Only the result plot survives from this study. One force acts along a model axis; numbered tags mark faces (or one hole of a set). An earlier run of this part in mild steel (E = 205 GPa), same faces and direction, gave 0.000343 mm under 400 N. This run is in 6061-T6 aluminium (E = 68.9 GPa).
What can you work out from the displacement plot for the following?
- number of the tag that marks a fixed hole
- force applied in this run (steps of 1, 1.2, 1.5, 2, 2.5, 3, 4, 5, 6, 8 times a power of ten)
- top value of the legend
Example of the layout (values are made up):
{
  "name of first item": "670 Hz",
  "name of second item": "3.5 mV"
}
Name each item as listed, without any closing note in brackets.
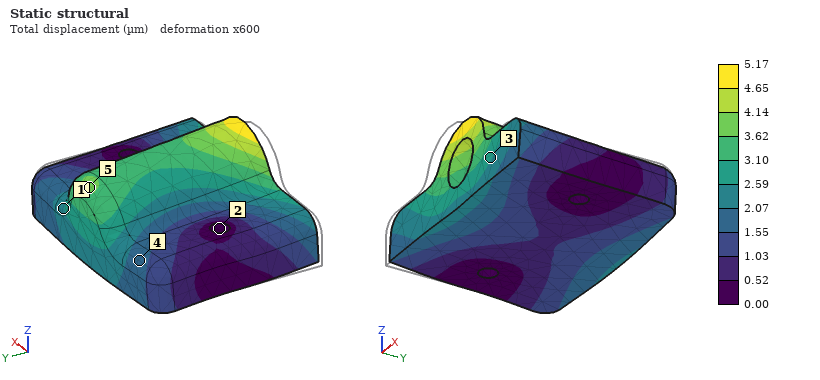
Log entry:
{
  "number of the tag that marks a fixed hole": "2",
  "force applied in this run": "2 kN",
  "top value of the legend": "5.17 µm"
}
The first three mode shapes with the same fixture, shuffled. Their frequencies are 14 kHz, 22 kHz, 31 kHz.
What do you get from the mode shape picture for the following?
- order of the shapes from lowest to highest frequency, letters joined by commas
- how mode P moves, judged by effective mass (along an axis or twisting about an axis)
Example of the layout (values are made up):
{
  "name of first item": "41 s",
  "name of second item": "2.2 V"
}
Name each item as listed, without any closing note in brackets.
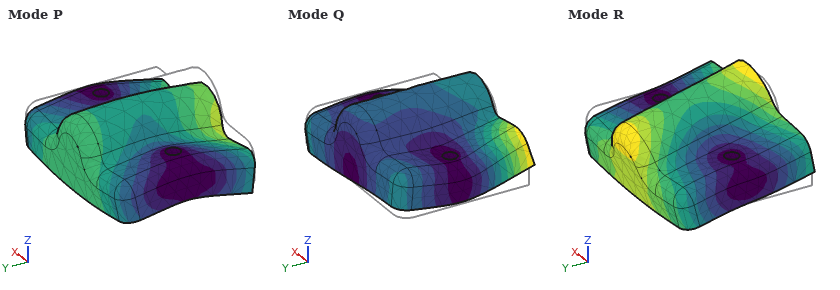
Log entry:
{
  "order of the shapes from lowest to highest frequency, letters joined by commas": "R, P, Q",
  "how mode P moves, judged by effective mass": "along Z"
}
